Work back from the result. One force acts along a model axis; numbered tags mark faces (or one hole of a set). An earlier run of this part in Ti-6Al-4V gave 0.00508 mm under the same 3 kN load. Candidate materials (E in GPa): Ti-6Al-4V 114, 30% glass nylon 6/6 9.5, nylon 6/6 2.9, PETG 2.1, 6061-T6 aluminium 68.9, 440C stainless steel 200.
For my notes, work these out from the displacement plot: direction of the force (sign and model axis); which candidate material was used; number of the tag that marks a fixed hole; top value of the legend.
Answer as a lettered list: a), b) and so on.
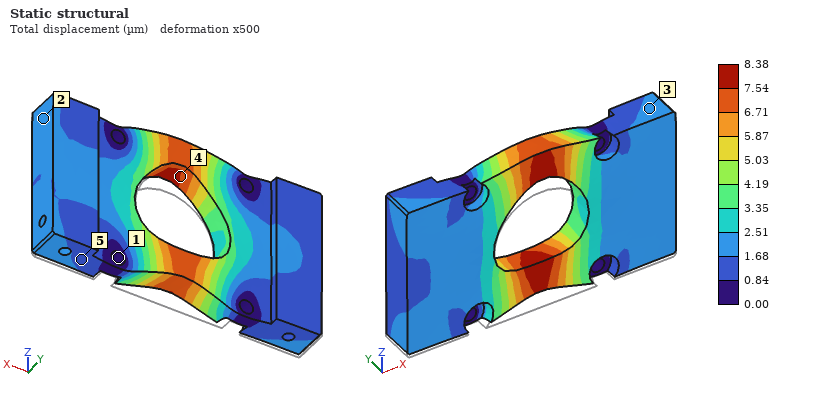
a) +Z
b) 6061-T6 aluminium
c) 1
d) 8.38 µm
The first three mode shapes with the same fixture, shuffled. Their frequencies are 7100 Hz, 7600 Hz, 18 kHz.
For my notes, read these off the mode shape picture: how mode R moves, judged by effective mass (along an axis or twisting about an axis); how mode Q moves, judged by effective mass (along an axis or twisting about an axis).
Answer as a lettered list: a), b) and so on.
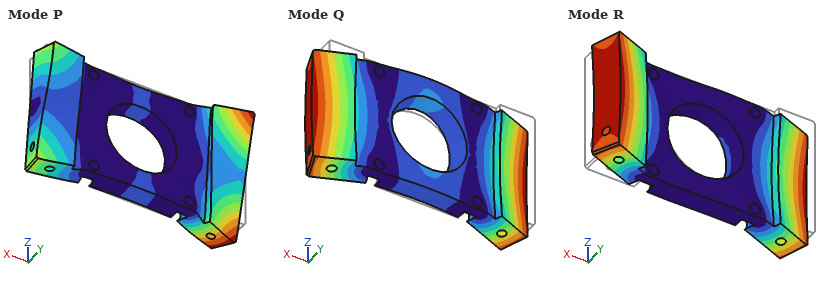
a) twisting about Z
b) along Y
